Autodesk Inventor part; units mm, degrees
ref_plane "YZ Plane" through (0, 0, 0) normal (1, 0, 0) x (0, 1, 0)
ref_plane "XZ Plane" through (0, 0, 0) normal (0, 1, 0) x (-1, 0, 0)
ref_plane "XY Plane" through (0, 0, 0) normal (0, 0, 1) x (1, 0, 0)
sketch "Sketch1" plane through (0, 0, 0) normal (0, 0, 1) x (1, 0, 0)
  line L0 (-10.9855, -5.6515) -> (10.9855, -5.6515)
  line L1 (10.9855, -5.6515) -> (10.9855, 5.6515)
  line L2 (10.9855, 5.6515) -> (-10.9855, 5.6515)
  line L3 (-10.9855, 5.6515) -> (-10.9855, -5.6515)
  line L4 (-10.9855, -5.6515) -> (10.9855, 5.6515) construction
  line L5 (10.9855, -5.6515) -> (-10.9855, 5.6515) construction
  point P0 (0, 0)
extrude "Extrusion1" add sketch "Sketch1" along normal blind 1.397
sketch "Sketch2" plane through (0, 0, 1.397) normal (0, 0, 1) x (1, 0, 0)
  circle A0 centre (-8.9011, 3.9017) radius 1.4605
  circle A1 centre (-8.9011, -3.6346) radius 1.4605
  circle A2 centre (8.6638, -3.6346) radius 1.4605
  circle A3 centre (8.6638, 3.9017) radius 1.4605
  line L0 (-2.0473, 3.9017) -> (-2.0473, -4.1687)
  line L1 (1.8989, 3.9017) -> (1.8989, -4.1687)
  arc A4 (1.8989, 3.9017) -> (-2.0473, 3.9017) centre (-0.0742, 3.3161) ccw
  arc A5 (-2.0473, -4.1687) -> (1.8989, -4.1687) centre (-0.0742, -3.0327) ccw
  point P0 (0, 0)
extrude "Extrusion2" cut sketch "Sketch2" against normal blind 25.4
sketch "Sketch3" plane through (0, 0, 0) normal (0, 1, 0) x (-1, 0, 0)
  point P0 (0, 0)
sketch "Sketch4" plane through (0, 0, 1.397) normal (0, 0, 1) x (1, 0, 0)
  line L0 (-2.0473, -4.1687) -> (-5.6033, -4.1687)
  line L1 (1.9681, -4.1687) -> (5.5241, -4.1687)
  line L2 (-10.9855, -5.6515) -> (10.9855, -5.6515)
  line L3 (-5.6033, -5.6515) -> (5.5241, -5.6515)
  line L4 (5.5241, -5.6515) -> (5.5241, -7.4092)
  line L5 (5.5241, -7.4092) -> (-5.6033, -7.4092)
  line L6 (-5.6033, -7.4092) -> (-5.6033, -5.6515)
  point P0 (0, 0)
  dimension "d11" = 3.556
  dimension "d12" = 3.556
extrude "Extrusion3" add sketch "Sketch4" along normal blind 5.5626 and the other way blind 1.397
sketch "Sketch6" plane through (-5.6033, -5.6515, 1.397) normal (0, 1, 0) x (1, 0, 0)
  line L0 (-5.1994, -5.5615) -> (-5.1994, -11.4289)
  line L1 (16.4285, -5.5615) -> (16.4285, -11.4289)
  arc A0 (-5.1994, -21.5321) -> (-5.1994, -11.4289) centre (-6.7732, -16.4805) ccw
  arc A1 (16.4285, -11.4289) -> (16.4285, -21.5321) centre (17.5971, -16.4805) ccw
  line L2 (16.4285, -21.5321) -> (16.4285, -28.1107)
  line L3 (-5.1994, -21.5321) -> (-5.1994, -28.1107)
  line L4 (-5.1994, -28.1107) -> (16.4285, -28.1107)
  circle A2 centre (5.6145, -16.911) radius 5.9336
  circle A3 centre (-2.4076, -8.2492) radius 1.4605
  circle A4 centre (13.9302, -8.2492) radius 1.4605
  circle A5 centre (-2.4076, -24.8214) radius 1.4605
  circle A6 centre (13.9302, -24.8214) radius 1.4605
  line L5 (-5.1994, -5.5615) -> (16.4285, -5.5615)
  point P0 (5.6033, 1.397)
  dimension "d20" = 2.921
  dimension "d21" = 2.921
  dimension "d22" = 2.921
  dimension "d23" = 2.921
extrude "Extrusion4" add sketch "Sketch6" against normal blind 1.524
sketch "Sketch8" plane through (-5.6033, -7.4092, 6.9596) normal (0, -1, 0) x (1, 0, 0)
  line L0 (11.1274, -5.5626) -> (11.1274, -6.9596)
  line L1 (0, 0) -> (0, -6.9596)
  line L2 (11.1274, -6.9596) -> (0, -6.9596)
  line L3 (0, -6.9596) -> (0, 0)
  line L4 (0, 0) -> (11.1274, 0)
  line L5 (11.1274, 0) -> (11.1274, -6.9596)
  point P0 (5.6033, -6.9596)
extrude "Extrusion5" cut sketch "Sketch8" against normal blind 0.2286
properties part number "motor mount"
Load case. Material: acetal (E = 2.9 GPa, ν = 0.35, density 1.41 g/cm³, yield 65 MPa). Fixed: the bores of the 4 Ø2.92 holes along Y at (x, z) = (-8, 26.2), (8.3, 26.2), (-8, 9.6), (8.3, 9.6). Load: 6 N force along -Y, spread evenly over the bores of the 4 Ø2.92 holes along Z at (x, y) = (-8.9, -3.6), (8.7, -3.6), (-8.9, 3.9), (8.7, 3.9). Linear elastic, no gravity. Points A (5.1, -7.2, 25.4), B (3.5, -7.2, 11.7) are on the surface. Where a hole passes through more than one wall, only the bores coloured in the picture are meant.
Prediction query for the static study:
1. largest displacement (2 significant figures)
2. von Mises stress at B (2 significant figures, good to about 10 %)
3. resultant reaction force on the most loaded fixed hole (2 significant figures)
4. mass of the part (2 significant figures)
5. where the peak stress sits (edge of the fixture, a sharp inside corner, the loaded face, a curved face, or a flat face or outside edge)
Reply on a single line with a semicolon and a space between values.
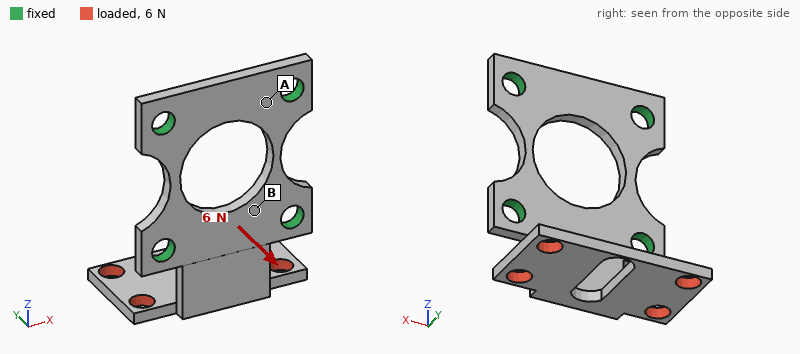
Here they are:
0.41 mm; 4.0 MPa; 3.4 N; 1.2 g; a flat face or outside edge
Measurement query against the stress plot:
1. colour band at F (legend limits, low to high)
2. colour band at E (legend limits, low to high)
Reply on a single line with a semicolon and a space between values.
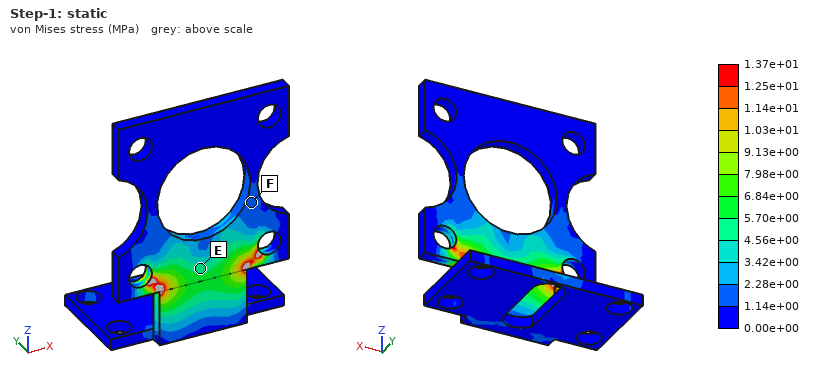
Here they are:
1.14e+00 to 2.28e+00 MPa; 4.56e+00 to 5.70e+00 MPa
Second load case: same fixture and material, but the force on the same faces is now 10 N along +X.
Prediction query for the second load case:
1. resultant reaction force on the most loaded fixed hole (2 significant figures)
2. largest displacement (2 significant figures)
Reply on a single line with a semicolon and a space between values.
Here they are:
9.9 N; 0.46 mm
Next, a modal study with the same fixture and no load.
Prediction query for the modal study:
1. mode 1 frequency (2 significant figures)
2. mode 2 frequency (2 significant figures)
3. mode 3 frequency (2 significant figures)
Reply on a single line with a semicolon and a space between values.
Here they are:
850 Hz; 1300 Hz; 2100 Hz
